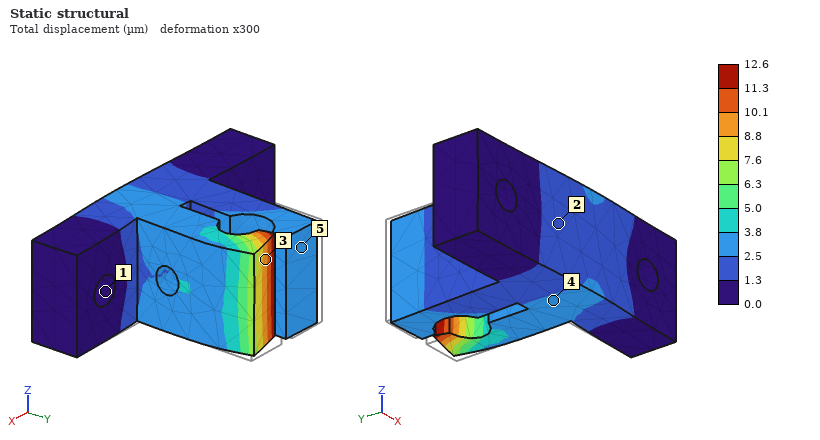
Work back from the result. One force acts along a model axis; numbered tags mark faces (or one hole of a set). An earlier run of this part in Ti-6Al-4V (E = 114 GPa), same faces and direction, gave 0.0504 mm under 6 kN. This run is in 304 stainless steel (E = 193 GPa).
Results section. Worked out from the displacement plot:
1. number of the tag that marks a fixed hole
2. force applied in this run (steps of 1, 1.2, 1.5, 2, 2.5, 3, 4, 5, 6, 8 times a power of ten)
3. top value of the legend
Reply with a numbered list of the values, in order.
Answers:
1. 1
2. 2.5 kN
3. 12.6 µm
